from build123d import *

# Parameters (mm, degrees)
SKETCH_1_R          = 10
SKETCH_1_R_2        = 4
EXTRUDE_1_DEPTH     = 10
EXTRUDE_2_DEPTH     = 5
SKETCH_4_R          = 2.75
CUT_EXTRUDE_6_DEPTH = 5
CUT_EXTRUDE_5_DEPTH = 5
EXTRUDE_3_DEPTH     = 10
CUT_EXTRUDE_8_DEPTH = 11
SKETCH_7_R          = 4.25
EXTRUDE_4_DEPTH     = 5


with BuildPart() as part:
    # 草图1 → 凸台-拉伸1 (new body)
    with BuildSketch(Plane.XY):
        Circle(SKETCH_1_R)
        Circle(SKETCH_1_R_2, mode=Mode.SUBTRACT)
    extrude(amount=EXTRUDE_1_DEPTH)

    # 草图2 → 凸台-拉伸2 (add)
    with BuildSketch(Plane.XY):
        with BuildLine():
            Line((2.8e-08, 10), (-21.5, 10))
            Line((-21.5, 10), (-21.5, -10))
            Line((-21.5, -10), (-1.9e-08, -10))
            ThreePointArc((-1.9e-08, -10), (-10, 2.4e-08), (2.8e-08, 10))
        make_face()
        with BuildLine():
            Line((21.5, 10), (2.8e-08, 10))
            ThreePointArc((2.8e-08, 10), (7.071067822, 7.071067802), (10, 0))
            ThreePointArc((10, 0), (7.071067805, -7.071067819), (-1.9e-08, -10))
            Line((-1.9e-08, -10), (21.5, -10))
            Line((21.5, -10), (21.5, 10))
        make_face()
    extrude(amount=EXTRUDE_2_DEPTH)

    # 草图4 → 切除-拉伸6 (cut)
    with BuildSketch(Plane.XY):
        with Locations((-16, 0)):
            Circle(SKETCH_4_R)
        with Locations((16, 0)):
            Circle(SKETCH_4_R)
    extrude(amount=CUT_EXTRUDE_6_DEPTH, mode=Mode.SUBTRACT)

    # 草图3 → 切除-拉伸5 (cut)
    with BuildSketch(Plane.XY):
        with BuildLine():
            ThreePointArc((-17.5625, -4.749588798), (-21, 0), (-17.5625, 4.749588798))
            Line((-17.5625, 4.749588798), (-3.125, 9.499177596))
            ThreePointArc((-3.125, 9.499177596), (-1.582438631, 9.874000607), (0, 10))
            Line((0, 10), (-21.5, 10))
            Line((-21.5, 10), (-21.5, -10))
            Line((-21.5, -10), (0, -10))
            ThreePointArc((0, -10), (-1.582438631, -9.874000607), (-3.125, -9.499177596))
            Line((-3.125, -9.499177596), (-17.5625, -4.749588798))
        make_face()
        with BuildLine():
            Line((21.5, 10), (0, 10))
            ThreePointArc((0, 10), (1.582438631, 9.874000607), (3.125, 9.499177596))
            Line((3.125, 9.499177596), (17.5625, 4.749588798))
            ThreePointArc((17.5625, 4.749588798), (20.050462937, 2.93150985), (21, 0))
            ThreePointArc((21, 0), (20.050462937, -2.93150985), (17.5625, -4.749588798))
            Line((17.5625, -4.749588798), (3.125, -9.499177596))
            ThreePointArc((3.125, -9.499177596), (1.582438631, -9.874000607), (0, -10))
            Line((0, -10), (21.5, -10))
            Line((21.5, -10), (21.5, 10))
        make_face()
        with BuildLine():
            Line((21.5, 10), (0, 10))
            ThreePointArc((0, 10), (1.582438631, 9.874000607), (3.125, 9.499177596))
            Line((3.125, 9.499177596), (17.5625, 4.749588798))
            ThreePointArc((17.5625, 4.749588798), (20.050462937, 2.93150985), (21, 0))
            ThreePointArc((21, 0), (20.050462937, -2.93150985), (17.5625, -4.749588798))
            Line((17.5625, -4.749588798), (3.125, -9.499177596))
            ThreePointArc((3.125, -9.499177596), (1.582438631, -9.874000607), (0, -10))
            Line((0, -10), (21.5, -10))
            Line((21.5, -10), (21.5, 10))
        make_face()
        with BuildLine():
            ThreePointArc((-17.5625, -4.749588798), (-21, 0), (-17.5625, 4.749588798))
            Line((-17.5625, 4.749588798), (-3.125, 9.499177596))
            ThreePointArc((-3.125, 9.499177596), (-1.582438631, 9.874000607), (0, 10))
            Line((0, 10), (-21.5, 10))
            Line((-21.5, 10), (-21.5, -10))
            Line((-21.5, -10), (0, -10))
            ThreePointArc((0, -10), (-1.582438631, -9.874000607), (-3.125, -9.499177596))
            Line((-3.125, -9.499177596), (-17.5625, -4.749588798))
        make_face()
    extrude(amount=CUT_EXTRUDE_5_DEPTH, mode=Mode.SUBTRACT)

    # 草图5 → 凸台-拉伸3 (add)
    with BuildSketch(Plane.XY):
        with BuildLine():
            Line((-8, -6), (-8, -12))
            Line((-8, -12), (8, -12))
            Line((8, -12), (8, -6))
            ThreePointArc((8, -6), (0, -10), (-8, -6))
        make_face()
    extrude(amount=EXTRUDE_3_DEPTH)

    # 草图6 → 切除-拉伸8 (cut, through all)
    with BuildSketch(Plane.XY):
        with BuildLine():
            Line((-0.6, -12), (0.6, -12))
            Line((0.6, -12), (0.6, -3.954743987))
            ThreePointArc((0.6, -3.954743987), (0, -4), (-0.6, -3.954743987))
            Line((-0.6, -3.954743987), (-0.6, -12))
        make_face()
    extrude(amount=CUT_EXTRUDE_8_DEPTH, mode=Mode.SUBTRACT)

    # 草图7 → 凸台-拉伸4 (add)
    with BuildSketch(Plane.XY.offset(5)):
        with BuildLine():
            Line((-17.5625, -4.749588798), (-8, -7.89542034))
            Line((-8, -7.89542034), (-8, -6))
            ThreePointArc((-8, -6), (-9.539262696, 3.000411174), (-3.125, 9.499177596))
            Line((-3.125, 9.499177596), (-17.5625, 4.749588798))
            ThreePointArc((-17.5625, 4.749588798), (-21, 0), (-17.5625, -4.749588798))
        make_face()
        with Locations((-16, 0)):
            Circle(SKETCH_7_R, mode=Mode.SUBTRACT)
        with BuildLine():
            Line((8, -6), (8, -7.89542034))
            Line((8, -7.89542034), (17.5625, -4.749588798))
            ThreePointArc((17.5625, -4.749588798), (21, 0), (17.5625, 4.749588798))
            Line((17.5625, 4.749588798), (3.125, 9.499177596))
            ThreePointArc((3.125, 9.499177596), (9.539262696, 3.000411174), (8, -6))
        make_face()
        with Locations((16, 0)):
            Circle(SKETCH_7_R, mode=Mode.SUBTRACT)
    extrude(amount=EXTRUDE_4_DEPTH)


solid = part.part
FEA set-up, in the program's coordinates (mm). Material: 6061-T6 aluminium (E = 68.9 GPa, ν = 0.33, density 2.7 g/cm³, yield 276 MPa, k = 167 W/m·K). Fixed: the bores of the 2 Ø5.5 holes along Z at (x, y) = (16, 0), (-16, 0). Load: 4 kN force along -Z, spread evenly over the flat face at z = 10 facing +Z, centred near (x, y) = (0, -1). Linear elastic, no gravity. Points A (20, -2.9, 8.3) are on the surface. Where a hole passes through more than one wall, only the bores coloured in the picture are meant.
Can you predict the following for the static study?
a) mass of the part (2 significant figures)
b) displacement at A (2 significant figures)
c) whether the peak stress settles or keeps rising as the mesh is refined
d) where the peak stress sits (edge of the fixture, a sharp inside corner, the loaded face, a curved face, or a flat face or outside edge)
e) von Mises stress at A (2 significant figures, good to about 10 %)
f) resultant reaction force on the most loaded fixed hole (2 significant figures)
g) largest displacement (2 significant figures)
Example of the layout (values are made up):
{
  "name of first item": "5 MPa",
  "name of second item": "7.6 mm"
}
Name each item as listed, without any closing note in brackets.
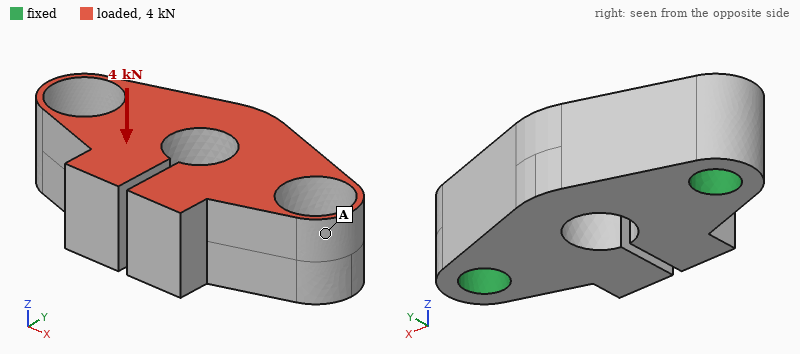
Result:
{
  "mass of the part": "13 g",
  "displacement at A": "10.0 µm",
  "whether the peak stress settles or keeps rising as the mesh is refined": "keeps rising",
  "where the peak stress sits": "edge of the fixture",
  "von Mises stress at A": "36 MPa",
  "resultant reaction force on the most loaded fixed hole": "2.1 kN",
  "largest displacement": "47 µm"
}
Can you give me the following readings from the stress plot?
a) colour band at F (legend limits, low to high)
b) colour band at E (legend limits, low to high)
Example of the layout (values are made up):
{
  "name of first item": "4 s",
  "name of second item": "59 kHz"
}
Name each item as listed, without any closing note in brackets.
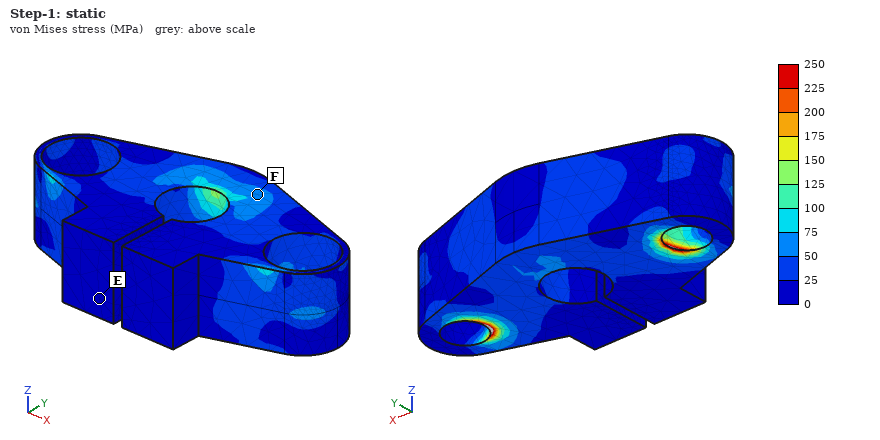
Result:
{
  "colour band at F": "50 to 75 MPa",
  "colour band at E": "0 to 25 MPa"
}
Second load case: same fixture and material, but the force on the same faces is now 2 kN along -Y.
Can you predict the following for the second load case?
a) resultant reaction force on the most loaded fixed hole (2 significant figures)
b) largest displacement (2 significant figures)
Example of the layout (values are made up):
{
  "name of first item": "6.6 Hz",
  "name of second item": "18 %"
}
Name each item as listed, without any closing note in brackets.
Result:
{
  "resultant reaction force on the most loaded fixed hole": "1.1 kN",
  "largest displacement": "34 µm"
}
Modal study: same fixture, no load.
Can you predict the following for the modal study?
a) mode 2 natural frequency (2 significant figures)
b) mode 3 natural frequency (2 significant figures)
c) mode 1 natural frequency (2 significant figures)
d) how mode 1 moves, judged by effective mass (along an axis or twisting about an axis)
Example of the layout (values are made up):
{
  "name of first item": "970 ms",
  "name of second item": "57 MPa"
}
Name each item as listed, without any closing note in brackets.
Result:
{
  "mode 2 natural frequency": "18 kHz",
  "mode 3 natural frequency": "19 kHz",
  "mode 1 natural frequency": "16 kHz",
  "how mode 1 moves, judged by effective mass": "along Z"
}
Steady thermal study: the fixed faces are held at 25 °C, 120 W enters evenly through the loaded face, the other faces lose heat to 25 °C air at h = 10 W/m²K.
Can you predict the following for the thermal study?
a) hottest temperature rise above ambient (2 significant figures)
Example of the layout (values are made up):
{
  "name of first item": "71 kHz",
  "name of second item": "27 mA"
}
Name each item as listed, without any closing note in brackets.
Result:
{
  "hottest temperature rise above ambient": "39 K"
}
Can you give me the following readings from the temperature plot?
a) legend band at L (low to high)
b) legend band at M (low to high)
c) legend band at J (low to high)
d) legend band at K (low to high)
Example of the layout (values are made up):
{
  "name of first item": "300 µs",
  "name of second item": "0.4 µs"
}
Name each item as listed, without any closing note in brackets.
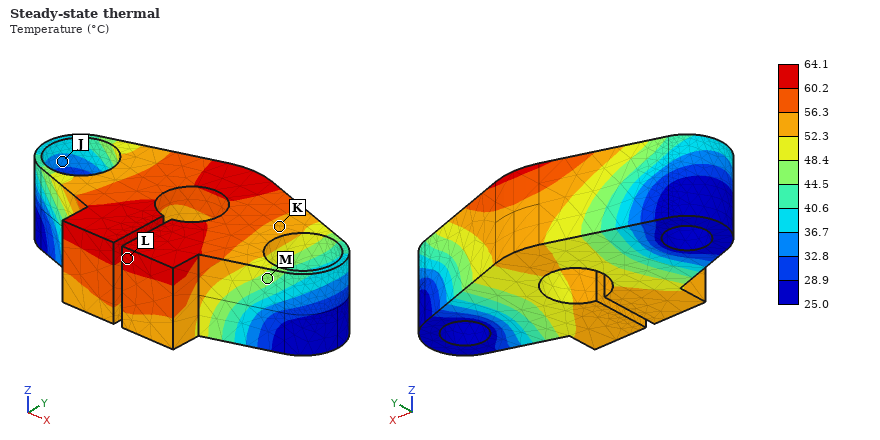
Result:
{
  "legend band at L": "60.2 to 64.1 °C",
  "legend band at M": "44.5 to 48.4 °C",
  "legend band at J": "32.8 to 36.7 °C",
  "legend band at K": "52.3 to 56.3 °C"
}
